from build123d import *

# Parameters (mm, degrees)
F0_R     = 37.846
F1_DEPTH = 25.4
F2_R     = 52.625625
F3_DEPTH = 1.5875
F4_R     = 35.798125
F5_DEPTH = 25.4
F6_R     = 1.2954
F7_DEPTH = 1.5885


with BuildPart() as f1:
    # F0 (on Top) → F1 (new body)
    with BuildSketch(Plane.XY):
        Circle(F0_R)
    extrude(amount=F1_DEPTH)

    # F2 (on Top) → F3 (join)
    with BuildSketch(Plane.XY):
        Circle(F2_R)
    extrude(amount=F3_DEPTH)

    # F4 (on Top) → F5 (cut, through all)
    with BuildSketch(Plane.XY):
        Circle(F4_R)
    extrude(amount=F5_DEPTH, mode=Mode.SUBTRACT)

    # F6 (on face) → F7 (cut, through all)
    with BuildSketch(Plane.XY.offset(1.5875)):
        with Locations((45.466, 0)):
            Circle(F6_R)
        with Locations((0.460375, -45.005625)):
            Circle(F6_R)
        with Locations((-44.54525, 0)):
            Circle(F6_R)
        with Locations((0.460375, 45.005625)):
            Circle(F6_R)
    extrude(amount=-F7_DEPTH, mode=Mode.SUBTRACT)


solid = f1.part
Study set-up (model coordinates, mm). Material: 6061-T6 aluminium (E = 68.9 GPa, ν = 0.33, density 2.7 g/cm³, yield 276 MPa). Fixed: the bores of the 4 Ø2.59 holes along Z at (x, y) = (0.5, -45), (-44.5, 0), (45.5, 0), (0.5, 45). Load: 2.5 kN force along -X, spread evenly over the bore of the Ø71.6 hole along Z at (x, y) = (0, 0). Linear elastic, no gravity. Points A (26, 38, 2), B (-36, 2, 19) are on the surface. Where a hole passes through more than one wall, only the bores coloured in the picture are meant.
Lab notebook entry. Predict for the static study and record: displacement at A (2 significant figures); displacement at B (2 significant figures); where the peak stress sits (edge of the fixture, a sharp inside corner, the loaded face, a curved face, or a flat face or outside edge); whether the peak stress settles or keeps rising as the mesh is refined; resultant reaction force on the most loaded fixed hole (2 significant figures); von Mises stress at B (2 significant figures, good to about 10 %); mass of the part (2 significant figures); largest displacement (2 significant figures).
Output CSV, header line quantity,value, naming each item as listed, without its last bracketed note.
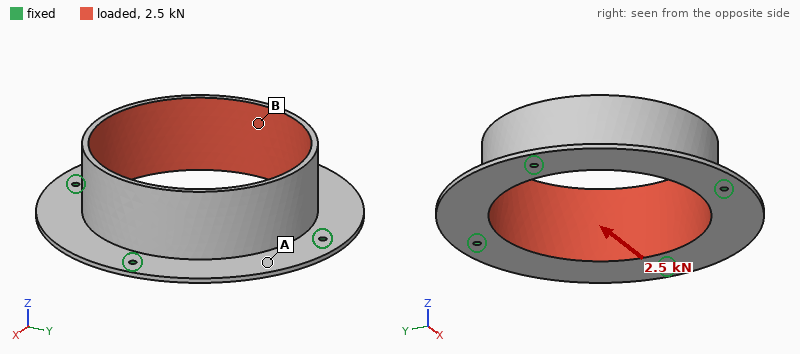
quantity,value
displacement at A,0.071 mm
displacement at B,0.049 mm
where the peak stress sits,edge of the fixture
whether the peak stress settles or keeps rising as the mesh is refined,keeps rising
resultant reaction force on the most loaded fixed hole,800 N
von Mises stress at B,35 MPa
mass of the part,50 g
largest displacement,0.11 mm
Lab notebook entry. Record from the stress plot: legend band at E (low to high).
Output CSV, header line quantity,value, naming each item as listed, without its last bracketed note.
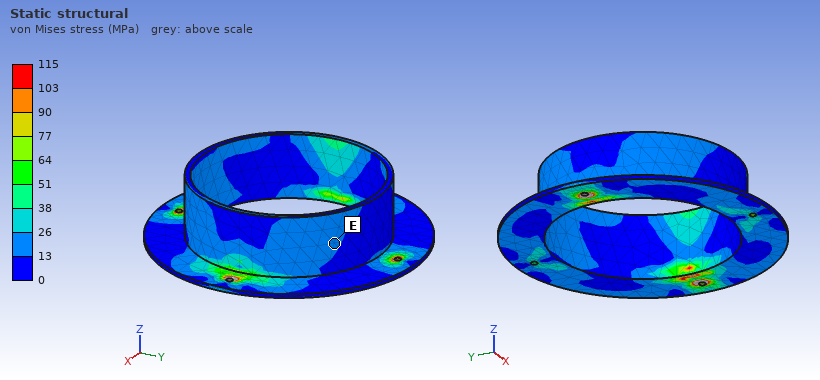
quantity,value
legend band at E,13 to 26 MPa
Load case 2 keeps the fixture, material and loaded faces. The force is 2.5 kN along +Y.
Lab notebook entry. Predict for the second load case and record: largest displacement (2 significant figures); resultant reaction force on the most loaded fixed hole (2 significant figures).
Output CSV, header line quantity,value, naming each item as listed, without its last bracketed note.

quantity,value
largest displacement,0.11 mm
resultant reaction force on the most loaded fixed hole,810 N
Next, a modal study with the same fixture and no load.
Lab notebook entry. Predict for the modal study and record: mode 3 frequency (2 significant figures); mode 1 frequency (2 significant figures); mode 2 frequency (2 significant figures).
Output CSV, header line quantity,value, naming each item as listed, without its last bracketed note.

quantity,value
mode 3 frequency,2600 Hz
mode 1 frequency,1700 Hz
mode 2 frequency,2600 Hz
